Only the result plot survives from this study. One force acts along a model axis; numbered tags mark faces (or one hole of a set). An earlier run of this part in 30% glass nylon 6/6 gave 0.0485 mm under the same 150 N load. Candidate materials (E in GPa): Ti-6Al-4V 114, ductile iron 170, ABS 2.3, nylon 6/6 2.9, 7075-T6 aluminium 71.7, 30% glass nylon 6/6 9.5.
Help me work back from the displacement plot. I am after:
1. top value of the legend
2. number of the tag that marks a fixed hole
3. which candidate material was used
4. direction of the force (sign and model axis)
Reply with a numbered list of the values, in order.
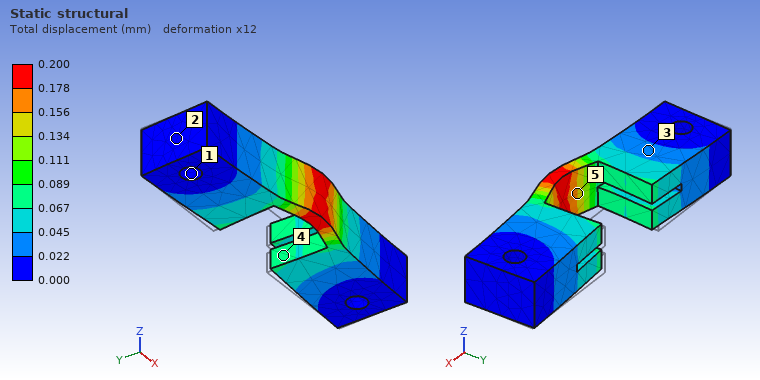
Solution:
1. 0.200 mm
2. 1
3. ABS
4. -Y
